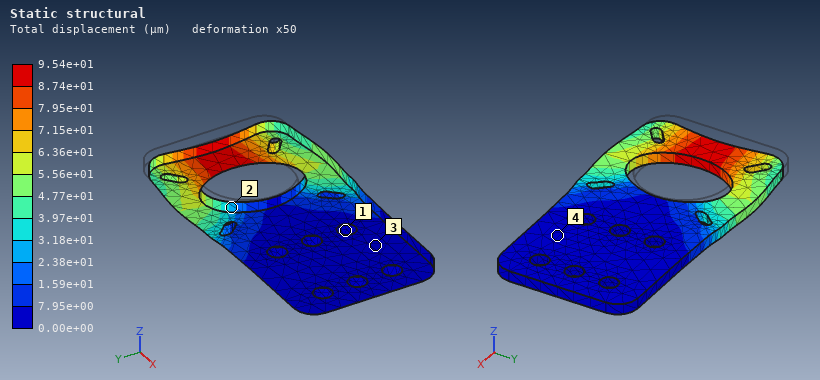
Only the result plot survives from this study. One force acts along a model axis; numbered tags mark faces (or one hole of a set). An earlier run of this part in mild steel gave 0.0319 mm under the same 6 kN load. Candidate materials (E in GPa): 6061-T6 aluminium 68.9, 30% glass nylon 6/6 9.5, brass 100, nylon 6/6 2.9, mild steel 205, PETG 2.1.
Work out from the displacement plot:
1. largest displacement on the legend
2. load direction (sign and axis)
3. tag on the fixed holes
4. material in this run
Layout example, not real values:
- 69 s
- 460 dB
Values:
- 9.54e+01 µm
- +X
- 1
- 6061-T6 aluminium
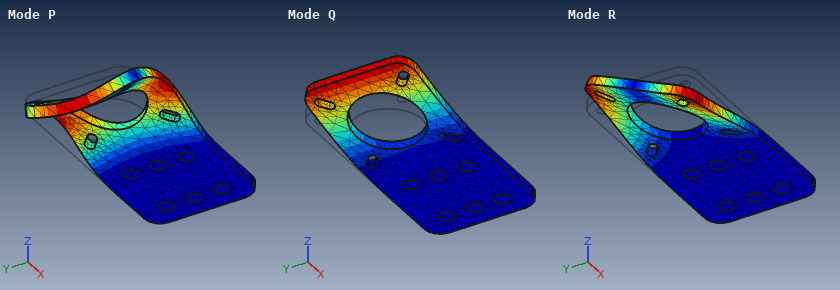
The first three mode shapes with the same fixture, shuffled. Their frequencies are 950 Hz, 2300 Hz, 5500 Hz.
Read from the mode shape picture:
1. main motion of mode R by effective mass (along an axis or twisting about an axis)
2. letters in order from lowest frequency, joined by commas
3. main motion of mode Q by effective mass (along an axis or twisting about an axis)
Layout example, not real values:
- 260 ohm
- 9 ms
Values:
- twisting about X
- Q, R, P
- along Z
